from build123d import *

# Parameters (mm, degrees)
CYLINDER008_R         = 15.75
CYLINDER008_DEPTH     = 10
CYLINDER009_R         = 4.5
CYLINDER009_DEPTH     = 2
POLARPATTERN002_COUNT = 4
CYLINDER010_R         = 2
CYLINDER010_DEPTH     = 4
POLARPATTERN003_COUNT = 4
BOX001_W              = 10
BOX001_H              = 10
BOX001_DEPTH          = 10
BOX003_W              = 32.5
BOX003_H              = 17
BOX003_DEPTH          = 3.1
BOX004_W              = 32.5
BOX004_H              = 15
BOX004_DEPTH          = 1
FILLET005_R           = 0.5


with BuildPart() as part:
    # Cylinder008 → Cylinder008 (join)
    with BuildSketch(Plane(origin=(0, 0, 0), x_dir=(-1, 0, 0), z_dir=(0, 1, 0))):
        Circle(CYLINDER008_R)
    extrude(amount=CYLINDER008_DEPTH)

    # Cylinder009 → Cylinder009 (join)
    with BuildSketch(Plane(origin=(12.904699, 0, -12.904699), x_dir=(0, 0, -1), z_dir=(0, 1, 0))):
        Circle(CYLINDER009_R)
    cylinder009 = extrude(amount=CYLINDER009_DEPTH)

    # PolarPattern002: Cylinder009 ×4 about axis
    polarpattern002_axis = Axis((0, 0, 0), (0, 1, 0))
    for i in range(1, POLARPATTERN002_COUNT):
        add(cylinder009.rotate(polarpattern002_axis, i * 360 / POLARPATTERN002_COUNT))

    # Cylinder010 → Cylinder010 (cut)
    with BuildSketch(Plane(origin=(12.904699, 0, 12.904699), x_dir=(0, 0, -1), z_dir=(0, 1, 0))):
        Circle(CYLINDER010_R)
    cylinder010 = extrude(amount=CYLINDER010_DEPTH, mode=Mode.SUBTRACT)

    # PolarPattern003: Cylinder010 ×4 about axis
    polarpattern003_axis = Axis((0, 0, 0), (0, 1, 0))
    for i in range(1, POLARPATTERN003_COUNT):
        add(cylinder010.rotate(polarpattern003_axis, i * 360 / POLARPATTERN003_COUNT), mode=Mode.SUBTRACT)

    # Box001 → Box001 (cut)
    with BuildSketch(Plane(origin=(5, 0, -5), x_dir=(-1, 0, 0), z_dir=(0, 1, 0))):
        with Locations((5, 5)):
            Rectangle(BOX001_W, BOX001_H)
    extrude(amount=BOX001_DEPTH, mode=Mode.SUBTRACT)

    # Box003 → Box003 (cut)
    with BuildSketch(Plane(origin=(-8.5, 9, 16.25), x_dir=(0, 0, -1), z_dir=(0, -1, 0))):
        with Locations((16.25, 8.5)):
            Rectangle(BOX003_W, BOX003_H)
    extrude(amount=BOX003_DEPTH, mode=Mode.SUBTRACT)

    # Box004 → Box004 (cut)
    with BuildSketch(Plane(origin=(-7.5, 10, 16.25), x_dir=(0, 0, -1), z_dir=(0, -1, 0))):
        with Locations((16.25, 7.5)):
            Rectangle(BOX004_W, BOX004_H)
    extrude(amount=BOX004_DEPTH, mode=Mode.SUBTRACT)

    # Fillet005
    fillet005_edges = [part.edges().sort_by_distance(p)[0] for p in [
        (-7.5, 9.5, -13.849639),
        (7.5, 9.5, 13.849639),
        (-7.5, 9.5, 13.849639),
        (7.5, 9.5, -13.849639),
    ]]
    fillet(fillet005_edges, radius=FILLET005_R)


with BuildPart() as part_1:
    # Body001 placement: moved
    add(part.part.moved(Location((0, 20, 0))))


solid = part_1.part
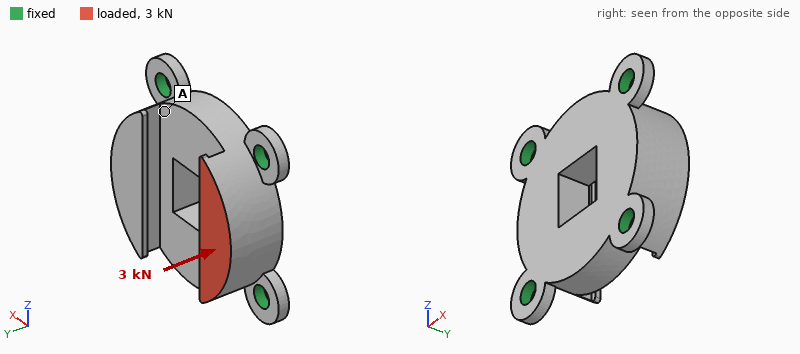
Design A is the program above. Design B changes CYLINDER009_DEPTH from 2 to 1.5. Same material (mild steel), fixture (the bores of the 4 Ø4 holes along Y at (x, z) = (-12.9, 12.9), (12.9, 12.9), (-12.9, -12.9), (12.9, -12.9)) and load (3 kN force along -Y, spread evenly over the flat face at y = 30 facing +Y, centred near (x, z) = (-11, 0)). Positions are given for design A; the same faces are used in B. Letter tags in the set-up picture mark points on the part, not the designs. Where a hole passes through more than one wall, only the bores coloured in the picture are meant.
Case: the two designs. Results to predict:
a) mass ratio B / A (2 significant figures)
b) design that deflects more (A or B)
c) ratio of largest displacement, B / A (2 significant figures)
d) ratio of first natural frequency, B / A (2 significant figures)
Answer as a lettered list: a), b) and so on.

a) 0.98
b) B
c) 1.2
d) 0.93
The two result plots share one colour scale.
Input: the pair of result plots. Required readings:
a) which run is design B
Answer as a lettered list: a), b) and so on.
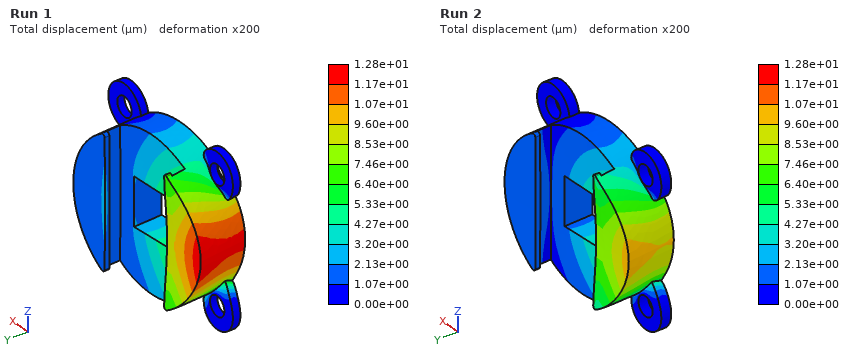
a) Run 1
